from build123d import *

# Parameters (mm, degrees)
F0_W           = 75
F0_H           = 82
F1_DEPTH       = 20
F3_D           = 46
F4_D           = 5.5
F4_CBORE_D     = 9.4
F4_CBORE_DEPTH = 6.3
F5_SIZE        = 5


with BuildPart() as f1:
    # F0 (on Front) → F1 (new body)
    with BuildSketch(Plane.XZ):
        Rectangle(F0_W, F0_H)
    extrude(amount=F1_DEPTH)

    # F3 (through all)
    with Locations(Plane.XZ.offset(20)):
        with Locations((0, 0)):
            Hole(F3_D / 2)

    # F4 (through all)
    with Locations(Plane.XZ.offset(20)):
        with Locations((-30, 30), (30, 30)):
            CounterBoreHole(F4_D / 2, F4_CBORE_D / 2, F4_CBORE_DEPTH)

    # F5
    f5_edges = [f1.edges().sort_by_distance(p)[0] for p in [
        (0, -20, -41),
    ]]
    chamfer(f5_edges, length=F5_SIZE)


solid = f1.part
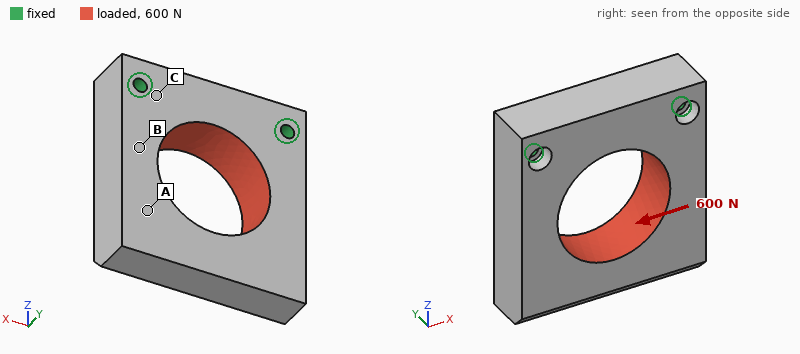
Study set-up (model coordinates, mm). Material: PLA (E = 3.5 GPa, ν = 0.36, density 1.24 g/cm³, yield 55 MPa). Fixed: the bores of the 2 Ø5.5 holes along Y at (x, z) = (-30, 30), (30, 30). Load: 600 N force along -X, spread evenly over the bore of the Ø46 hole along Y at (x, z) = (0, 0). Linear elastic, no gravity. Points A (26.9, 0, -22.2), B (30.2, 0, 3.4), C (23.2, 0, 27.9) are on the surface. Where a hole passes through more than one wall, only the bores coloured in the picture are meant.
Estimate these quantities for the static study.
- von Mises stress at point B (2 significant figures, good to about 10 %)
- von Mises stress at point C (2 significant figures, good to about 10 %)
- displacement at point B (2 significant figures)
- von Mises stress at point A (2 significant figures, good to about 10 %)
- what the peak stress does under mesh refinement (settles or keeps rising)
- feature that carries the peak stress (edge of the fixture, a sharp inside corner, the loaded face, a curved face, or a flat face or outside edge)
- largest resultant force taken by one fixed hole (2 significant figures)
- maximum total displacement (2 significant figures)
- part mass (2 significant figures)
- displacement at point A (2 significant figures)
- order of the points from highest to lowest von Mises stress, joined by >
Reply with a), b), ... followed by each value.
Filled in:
a) 1.9 MPa
b) 1.2 MPa
c) 40 µm
d) 0.49 MPa
e) keeps rising
f) edge of the fixture
g) 400 N
h) 88 µm
i) 110 g
j) 79 µm
k) B > C > A
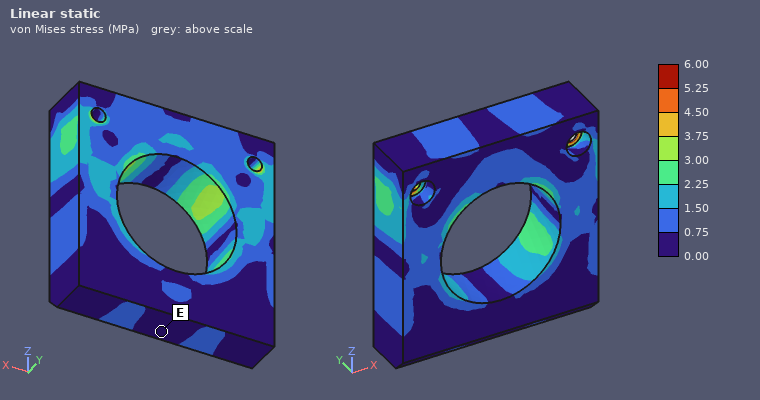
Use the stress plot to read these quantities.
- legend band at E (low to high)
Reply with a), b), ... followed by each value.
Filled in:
a) 0.00 to 0.75 MPa
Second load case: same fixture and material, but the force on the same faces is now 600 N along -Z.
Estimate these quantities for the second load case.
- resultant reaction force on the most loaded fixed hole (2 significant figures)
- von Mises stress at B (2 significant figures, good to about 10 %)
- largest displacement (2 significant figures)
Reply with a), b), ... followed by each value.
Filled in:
a) 300 N
b) 0.73 MPa
c) 29 µm
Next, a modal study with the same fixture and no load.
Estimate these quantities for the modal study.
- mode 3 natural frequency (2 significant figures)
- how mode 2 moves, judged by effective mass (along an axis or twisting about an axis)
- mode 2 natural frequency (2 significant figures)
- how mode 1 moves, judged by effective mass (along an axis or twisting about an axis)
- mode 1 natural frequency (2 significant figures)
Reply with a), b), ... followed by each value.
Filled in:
a) 1500 Hz
b) along X
c) 1400 Hz
d) along Y
e) 630 Hz
